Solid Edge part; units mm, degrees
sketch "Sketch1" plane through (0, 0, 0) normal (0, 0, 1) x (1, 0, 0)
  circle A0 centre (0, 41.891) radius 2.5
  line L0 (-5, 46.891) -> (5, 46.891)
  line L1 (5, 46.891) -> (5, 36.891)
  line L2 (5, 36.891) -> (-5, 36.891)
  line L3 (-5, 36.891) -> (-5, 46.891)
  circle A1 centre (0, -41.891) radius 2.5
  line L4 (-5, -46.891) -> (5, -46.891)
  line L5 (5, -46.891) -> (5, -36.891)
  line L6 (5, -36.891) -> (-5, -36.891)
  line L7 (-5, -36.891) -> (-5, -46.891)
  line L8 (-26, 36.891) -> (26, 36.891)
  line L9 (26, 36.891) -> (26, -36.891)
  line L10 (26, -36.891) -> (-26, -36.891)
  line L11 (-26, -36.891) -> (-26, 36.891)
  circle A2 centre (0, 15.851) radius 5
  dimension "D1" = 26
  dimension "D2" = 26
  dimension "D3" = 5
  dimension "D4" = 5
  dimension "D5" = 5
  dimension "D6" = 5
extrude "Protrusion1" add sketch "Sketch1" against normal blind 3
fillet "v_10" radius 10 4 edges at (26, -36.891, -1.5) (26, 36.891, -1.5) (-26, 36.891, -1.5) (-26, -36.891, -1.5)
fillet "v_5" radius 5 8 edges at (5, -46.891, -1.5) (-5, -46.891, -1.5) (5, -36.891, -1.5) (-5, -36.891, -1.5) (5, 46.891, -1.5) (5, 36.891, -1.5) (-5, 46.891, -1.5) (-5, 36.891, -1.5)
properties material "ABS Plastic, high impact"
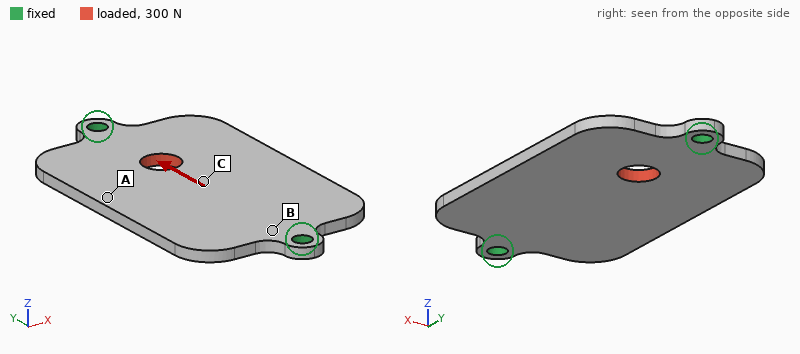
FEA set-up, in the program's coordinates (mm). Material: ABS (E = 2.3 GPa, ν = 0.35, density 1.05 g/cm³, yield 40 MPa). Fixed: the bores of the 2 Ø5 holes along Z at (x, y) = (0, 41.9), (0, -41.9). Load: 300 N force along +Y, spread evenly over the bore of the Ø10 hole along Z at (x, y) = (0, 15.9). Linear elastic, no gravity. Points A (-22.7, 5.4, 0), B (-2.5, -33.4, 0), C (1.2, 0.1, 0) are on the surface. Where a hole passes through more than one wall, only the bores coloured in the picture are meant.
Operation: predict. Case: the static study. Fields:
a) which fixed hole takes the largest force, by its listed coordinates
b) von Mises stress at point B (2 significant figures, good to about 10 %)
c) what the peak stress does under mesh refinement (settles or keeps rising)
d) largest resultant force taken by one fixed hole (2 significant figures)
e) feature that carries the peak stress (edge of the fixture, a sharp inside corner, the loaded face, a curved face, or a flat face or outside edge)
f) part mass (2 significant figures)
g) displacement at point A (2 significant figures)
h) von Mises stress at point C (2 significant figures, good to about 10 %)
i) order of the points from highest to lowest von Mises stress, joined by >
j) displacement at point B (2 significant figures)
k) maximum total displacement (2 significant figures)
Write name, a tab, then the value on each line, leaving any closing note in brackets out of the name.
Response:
which fixed hole takes the largest force, by its listed coordinates	(0, 41.9)
von Mises stress at point B	2.6 MPa
what the peak stress does under mesh refinement	keeps rising
largest resultant force taken by one fixed hole	180 N
feature that carries the peak stress	edge of the fixture
part mass	12 g
displacement at point A	26 µm
von Mises stress at point C	1.9 MPa
order of the points from highest to lowest von Mises stress, joined by >	B > C > A
displacement at point B	9.7 µm
maximum total displacement	46 µm
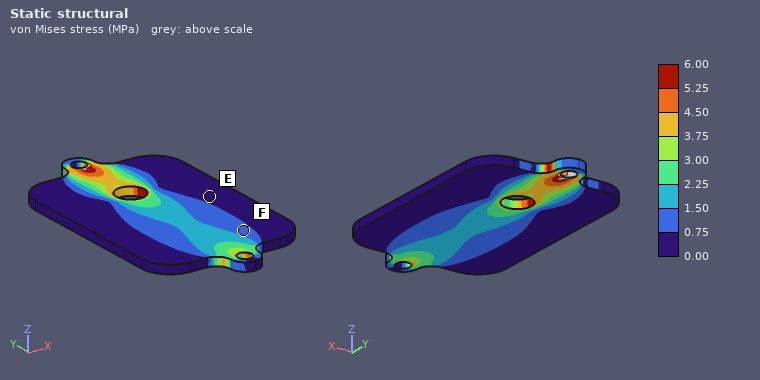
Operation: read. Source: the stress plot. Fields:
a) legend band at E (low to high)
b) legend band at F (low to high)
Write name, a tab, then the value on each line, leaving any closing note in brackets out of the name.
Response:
legend band at E	0.00 to 0.75 MPa
legend band at F	0.75 to 1.50 MPa
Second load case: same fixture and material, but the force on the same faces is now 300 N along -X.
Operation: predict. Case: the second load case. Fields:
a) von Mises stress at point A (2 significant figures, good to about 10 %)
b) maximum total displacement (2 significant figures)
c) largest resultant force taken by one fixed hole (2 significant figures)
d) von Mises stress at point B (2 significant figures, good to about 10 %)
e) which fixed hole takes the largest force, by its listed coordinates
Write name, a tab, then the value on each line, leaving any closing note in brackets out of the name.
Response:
von Mises stress at point A	2.8 MPa
maximum total displacement	0.11 mm
largest resultant force taken by one fixed hole	210 N
von Mises stress at point B	1.8 MPa
which fixed hole takes the largest force, by its listed coordinates	(0, 41.9)
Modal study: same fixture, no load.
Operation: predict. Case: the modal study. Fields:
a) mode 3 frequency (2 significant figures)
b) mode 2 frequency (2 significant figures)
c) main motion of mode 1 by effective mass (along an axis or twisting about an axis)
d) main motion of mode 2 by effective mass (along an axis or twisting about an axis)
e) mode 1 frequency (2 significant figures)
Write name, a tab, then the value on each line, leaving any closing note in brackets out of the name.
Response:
mode 3 frequency	1100 Hz
mode 2 frequency	470 Hz
main motion of mode 1 by effective mass	twisting about Y
main motion of mode 2 by effective mass	along Z
mode 1 frequency	420 Hz
